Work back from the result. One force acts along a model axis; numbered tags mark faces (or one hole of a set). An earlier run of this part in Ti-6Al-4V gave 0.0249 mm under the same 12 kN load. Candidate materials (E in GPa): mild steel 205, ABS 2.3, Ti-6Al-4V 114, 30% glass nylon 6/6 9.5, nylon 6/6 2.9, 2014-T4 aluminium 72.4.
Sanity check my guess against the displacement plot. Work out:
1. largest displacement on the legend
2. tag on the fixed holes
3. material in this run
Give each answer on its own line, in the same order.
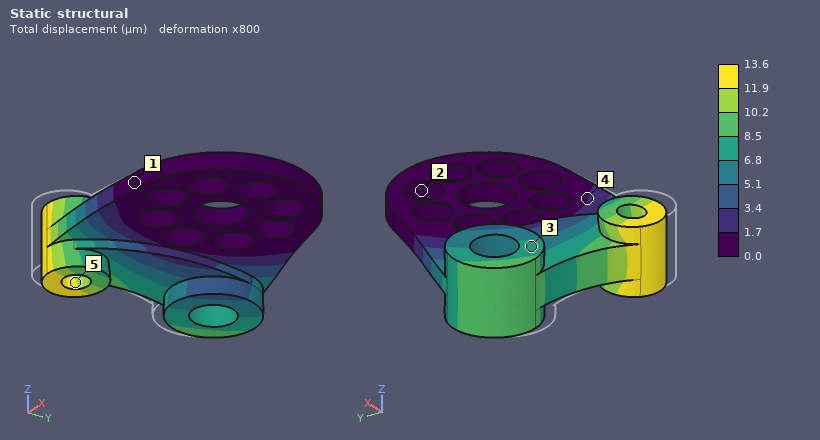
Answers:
13.6 µm
2
mild steel
